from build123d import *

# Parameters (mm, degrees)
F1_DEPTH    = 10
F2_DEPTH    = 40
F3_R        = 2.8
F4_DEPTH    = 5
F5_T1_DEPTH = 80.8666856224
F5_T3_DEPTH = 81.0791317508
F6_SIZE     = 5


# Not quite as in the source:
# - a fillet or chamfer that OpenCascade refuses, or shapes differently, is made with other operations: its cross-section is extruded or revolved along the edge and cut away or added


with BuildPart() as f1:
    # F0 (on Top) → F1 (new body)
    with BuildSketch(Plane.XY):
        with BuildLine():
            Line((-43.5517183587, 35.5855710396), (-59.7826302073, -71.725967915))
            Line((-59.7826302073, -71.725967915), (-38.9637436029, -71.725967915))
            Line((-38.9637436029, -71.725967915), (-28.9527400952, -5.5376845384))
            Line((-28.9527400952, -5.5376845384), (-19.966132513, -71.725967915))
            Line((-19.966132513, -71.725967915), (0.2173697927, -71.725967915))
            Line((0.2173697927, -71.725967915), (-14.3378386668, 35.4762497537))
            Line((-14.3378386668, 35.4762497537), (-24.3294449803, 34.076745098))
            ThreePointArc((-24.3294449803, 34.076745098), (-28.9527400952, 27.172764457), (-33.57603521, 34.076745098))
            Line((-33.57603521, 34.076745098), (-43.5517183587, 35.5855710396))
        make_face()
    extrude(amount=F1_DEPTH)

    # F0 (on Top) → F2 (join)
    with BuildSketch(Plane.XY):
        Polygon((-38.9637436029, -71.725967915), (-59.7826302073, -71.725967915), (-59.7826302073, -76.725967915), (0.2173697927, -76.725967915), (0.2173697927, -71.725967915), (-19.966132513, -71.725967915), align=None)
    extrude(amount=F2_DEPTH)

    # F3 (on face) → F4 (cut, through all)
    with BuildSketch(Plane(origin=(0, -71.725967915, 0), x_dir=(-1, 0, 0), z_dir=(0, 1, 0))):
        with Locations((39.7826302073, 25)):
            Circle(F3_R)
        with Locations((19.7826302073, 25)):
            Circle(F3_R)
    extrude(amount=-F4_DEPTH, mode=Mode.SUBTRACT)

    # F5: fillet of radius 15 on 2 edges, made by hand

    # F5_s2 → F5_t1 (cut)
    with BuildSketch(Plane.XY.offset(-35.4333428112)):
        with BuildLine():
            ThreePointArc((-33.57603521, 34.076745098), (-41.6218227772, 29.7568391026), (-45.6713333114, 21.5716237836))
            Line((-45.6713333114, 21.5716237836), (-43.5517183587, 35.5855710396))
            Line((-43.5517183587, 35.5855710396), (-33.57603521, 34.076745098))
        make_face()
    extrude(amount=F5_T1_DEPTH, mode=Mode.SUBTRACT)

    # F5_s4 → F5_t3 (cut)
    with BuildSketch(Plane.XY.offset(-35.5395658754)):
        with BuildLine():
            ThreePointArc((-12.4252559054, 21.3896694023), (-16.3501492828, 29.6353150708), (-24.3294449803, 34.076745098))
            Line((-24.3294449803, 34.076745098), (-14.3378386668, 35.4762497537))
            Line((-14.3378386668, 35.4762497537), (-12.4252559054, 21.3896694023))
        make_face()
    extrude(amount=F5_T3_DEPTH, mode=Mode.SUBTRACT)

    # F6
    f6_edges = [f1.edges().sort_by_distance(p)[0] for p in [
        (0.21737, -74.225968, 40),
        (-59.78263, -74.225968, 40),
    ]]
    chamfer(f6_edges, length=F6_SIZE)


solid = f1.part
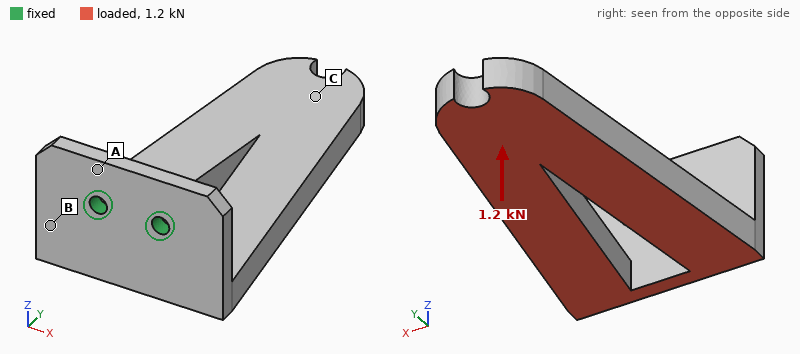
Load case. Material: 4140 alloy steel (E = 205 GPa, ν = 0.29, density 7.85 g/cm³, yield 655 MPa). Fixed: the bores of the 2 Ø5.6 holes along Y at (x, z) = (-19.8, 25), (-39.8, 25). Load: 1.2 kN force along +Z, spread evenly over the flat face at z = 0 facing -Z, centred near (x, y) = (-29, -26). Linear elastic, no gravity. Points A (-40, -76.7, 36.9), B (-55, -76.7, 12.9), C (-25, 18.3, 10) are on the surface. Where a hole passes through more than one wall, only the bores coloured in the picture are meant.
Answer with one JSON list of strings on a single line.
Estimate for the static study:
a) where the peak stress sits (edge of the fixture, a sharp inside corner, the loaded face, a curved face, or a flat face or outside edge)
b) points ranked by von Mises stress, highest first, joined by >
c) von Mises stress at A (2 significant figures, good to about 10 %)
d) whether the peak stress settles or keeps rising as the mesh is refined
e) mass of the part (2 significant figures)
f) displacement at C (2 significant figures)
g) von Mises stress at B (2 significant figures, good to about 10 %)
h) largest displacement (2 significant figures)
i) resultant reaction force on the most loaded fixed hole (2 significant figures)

["edge of the fixture", "B > A > C", "52 MPa", "keeps rising", "400 g", "0.94 mm", "210 MPa", "1.1 mm", "610 N"]
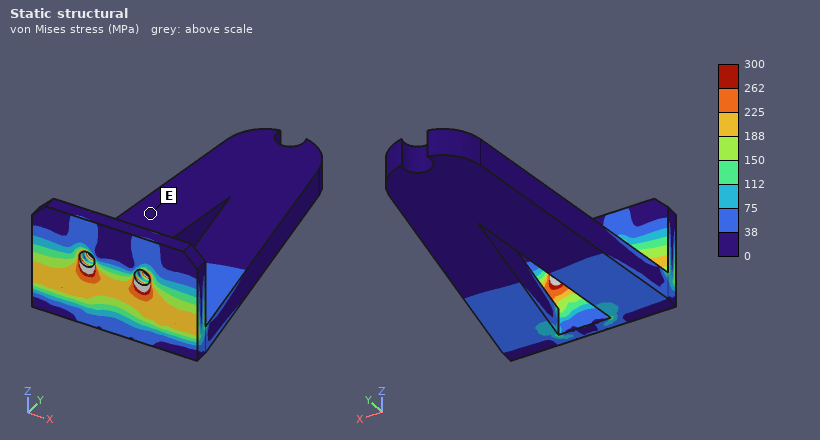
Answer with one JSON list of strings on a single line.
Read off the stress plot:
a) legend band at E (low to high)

["0 to 38 MPa"]
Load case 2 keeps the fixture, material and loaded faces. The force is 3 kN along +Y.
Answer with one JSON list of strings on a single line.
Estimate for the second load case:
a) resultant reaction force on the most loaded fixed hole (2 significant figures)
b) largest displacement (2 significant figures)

["1.5 kN", "0.83 mm"]
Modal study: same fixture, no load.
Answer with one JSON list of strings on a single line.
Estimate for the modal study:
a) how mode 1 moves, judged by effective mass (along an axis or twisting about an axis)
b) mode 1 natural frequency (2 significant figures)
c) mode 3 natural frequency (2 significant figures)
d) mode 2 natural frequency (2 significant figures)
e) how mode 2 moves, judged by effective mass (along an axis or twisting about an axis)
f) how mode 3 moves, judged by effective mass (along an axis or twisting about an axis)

["along Z", "360 Hz", "2600 Hz", "770 Hz", "along X", "along Y"]
